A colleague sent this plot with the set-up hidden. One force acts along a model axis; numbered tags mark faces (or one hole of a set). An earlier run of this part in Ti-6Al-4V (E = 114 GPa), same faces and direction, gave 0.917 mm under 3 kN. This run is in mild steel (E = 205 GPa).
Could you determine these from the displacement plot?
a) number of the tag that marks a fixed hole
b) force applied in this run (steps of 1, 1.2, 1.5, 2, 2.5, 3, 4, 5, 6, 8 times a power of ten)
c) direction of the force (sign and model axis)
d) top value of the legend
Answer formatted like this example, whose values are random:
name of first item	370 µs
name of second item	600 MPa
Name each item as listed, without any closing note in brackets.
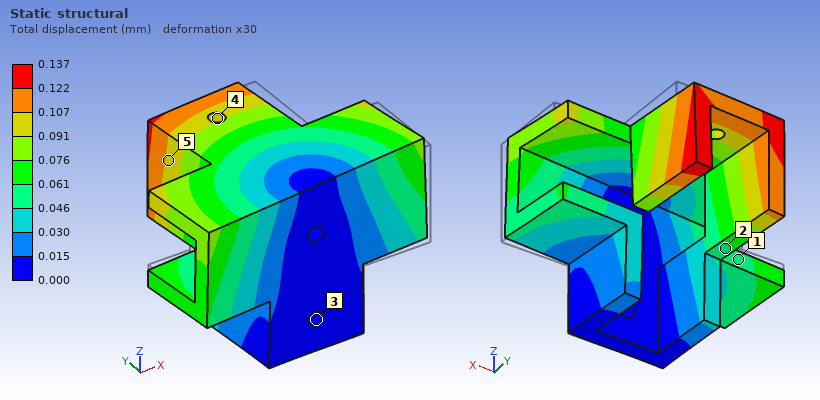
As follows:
number of the tag that marks a fixed hole	3
force applied in this run	800 N
direction of the force	-X
top value of the legend	0.137 mm
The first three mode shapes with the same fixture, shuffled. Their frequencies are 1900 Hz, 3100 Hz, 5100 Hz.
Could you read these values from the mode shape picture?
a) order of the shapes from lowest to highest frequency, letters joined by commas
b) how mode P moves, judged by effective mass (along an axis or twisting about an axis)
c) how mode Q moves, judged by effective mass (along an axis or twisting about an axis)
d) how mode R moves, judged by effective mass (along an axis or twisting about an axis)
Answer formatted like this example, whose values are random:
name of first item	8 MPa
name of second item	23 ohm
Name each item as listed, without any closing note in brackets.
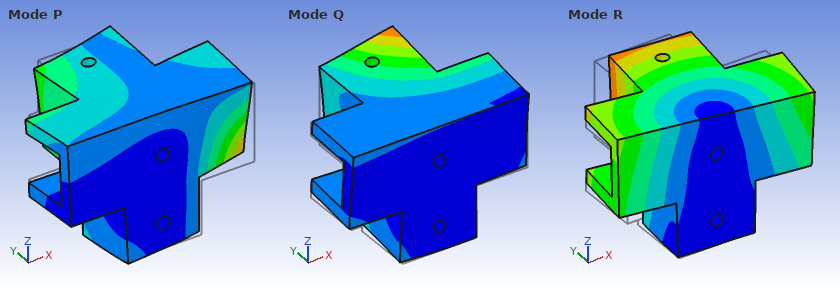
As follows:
order of the shapes from lowest to highest frequency, letters joined by commas	R, Q, P
how mode P moves, judged by effective mass	along Y
how mode Q moves, judged by effective mass	along Z
how mode R moves, judged by effective mass	along X
